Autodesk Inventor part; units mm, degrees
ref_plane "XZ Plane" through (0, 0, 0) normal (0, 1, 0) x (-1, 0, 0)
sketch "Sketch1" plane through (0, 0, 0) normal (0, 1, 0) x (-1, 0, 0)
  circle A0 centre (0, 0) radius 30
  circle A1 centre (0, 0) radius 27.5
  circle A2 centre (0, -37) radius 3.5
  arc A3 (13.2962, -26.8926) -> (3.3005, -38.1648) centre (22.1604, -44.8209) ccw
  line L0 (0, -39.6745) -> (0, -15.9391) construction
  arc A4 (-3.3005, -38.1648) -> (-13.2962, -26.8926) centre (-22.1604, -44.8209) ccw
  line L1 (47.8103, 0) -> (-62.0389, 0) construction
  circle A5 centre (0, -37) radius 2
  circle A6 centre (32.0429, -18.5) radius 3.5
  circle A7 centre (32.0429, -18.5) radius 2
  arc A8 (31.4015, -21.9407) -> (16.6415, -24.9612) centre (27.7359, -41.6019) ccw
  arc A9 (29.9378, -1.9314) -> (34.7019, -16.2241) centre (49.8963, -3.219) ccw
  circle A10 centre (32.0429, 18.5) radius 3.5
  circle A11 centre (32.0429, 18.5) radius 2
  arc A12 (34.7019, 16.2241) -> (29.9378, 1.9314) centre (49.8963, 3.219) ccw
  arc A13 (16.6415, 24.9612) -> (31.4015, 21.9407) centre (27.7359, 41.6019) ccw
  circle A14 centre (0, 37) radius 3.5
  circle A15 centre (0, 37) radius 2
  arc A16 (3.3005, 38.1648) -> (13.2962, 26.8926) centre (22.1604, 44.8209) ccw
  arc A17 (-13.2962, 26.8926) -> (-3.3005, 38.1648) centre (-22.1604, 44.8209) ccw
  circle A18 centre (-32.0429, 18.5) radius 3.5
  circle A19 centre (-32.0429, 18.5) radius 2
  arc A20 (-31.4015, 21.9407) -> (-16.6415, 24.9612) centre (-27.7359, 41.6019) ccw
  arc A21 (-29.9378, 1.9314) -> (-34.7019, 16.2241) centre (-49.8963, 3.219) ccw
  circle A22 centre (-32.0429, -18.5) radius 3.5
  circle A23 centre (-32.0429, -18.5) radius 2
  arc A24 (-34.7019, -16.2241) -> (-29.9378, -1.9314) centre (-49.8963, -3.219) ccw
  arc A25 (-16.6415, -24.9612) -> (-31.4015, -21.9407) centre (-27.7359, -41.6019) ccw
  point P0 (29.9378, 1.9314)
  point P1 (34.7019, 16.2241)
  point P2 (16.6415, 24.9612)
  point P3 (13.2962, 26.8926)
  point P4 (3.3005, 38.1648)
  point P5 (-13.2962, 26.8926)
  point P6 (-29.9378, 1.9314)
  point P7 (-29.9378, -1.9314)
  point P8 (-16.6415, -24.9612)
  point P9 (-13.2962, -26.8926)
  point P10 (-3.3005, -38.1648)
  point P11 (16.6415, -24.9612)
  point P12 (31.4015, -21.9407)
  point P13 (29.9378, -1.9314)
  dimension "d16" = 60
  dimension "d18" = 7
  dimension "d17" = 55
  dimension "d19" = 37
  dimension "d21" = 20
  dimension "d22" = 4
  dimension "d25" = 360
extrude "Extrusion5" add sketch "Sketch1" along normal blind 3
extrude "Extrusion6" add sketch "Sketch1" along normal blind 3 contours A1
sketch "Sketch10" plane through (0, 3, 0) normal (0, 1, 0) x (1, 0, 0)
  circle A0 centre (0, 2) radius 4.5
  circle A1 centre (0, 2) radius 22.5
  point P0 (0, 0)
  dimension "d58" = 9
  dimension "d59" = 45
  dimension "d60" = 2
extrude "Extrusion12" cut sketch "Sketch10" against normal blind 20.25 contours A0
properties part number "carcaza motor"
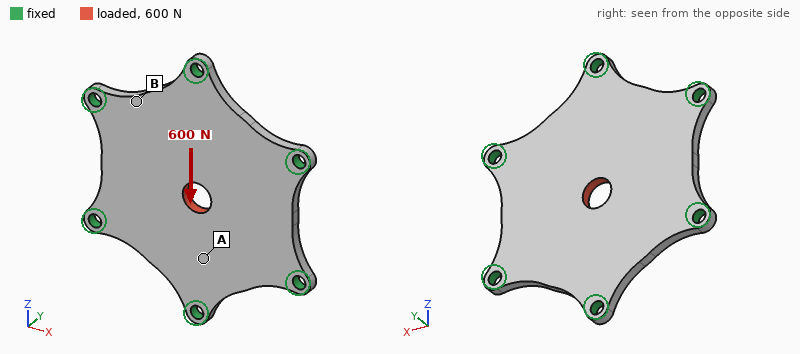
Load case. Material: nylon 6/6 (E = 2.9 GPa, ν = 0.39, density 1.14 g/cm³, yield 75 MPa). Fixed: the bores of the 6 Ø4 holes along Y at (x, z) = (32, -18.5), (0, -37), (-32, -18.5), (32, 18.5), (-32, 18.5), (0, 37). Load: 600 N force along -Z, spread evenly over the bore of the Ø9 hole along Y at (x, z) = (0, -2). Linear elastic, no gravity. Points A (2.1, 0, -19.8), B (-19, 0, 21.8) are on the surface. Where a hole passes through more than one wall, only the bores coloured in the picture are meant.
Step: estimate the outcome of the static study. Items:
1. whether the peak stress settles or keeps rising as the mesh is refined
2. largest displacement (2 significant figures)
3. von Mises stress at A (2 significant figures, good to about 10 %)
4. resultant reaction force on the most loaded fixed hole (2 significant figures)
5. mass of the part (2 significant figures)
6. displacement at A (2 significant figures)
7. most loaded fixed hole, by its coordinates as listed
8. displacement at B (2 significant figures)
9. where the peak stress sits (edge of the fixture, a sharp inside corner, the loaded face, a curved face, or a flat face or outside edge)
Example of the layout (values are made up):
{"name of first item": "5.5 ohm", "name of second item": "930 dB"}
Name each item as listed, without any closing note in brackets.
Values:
{"whether the peak stress settles or keeps rising as the mesh is refined": "keeps rising", "largest displacement": "54 µm", "von Mises stress at A": "4.4 MPa", "resultant reaction force on the most loaded fixed hole": "180 N", "mass of the part": "12 g", "displacement at A": "29 µm", "most loaded fixed hole, by its coordinates as listed": "(0, -37)", "displacement at B": "22 µm", "where the peak stress sits": "edge of the fixture"}
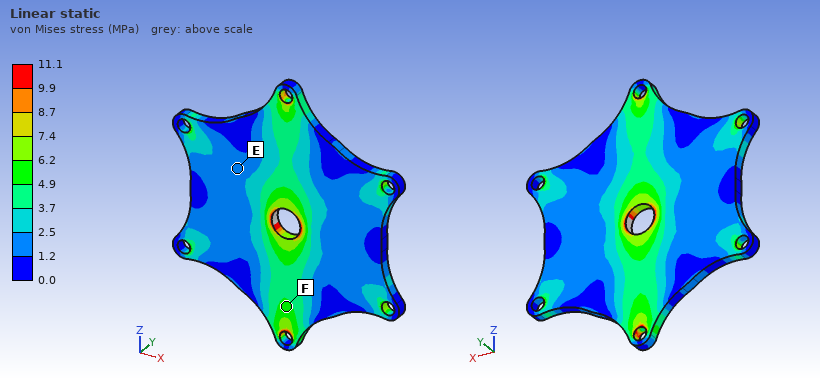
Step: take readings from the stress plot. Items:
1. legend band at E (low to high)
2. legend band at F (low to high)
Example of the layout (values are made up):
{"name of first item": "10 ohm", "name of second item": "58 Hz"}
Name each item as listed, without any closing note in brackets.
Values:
{"legend band at E": "1.2 to 2.5 MPa", "legend band at F": "4.9 to 6.2 MPa"}
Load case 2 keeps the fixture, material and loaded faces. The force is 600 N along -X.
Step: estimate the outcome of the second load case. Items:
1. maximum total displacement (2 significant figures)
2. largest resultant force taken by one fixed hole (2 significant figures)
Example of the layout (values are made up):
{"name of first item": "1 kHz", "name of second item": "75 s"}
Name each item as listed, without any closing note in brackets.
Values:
{"maximum total displacement": "54 µm", "largest resultant force taken by one fixed hole": "160 N"}
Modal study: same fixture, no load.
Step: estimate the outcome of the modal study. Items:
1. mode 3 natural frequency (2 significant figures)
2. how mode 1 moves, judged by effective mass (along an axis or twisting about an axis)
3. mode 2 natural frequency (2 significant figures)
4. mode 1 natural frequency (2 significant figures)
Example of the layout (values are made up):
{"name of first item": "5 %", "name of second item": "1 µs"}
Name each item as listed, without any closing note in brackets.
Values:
{"mode 3 natural frequency": "2800 Hz", "how mode 1 moves, judged by effective mass": "along Y", "mode 2 natural frequency": "2800 Hz", "mode 1 natural frequency": "1300 Hz"}
